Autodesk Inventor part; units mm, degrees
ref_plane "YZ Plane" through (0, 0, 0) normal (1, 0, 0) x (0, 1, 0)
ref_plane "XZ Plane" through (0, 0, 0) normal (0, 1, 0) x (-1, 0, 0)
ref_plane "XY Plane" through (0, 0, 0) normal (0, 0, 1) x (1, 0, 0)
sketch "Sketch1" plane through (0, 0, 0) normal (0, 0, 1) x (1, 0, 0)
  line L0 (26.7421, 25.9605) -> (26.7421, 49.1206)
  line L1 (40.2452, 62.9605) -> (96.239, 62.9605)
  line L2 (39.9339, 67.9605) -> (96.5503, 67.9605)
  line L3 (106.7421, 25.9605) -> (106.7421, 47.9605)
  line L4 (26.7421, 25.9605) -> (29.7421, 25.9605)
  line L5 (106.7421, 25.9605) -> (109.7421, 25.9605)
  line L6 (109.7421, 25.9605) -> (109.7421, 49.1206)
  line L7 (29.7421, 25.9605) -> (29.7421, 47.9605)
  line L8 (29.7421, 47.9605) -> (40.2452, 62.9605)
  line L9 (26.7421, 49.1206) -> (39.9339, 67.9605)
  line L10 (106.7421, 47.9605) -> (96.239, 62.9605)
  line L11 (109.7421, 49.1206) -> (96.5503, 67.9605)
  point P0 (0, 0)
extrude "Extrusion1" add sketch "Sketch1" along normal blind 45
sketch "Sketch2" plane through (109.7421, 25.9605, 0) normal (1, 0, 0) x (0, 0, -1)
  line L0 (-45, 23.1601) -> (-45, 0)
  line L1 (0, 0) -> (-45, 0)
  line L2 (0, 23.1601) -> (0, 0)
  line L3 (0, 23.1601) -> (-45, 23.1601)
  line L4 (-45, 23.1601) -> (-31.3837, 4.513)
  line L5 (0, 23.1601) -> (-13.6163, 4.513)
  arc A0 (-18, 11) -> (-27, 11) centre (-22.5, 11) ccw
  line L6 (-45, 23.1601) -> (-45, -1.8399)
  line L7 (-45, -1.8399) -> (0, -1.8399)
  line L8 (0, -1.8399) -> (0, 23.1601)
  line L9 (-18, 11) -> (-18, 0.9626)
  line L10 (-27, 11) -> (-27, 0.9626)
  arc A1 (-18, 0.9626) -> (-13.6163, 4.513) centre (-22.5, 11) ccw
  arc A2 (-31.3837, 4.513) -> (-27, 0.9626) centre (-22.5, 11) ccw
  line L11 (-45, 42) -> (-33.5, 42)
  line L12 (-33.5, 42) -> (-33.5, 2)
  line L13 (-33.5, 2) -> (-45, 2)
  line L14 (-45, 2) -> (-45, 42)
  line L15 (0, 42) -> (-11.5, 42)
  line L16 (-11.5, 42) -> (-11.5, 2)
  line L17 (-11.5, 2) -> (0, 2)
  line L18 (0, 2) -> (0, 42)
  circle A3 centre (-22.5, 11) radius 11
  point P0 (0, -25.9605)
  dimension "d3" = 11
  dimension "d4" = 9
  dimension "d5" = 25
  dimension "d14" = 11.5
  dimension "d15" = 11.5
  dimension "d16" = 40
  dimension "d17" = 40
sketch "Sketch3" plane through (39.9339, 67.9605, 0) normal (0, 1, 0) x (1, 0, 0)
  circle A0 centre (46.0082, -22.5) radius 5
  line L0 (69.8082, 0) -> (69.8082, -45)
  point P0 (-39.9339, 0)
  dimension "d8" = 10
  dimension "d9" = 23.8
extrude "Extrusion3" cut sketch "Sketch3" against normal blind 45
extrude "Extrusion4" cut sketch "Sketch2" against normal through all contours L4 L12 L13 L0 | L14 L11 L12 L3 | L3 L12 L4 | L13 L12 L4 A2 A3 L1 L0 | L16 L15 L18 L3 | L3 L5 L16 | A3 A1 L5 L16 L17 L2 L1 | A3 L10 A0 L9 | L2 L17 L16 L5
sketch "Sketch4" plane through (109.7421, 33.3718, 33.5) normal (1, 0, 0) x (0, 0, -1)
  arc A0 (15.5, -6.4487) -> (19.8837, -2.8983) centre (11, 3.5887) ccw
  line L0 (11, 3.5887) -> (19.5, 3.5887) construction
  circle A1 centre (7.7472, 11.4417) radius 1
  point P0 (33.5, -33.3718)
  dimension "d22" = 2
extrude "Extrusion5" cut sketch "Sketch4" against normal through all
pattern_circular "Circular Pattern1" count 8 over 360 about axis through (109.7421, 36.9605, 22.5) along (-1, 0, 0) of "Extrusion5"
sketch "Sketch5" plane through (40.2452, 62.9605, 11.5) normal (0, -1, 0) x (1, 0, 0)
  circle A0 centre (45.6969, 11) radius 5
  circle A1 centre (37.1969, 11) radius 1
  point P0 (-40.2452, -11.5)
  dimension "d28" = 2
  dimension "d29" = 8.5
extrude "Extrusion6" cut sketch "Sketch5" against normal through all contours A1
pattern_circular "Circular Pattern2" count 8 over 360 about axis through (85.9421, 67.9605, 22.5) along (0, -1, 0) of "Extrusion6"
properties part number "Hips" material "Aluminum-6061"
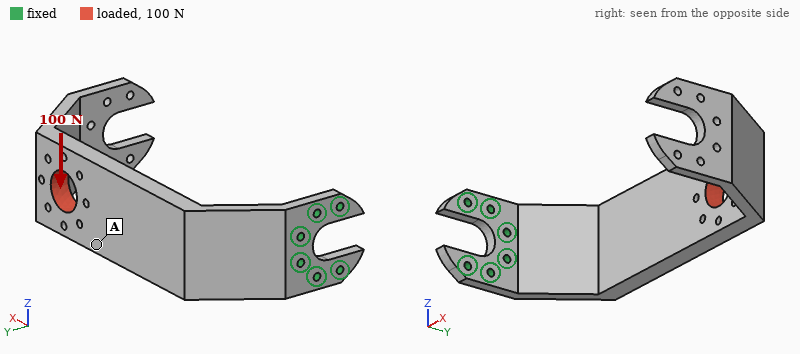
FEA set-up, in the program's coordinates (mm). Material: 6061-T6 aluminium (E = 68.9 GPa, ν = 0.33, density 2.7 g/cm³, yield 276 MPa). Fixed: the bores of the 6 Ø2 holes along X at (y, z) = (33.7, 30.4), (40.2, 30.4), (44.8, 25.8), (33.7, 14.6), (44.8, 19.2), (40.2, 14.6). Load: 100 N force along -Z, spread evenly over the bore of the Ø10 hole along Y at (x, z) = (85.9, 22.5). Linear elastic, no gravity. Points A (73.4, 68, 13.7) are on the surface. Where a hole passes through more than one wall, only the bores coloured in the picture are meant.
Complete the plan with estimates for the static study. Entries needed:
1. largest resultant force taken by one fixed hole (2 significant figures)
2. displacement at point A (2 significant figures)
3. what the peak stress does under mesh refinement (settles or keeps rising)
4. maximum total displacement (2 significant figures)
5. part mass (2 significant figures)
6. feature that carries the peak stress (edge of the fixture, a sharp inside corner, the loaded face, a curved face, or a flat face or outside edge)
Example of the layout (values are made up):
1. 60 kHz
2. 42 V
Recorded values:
1. 450 N
2. 0.42 mm
3. keeps rising
4. 1.1 mm
5. 28 g
6. edge of the fixture
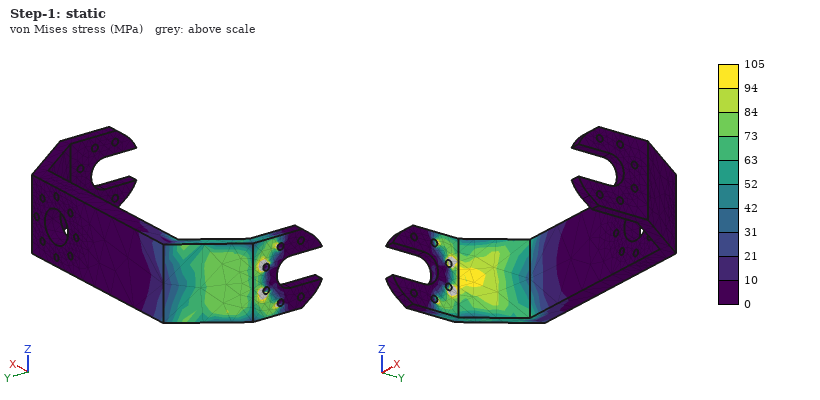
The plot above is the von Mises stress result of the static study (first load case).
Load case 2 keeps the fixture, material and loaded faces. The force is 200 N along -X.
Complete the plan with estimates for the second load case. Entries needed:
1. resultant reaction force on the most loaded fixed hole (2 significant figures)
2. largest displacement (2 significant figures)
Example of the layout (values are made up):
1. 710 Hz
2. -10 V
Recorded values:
1. 220 N
2. 1.0 mm
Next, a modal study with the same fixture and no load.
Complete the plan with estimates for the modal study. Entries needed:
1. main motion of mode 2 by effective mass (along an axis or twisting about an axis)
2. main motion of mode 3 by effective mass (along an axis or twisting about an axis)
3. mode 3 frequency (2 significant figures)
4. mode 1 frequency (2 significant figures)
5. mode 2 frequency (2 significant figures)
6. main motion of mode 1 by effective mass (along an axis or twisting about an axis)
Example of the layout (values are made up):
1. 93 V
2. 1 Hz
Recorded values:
1. along Z
2. along X
3. 1200 Hz
4. 260 Hz
5. 430 Hz
6. along Y
